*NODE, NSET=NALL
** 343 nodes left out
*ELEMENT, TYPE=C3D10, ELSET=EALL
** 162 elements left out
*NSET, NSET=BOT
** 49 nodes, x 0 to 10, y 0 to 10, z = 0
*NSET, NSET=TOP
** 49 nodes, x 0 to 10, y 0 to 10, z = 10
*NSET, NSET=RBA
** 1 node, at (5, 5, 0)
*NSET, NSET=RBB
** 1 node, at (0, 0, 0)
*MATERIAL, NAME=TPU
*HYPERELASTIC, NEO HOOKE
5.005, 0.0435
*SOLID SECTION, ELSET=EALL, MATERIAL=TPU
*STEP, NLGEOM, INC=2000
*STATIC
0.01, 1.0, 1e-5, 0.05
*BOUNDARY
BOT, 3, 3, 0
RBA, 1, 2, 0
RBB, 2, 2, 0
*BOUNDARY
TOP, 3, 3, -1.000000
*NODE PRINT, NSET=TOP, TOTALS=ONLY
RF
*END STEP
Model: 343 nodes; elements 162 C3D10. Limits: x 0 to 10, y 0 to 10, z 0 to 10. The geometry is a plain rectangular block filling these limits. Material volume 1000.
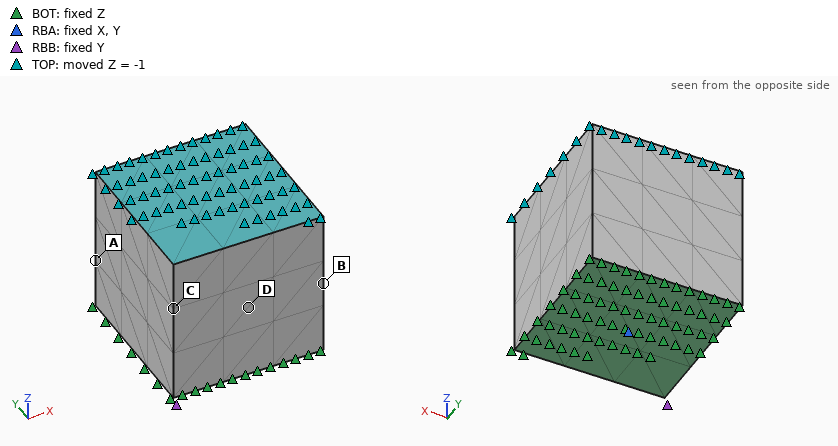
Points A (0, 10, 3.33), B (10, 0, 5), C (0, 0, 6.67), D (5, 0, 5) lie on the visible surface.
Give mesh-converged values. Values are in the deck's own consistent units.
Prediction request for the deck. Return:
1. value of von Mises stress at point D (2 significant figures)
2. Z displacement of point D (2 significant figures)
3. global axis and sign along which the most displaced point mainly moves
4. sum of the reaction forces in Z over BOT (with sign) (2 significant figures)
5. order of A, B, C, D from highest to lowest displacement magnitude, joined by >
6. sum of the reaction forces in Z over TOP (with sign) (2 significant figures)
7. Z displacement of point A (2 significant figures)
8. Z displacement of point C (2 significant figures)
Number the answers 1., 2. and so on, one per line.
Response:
1. 2.9
2. -0.50
3. -Z
4. 310
5. C > B > D > A
6. -310
7. -0.33
8. -0.67
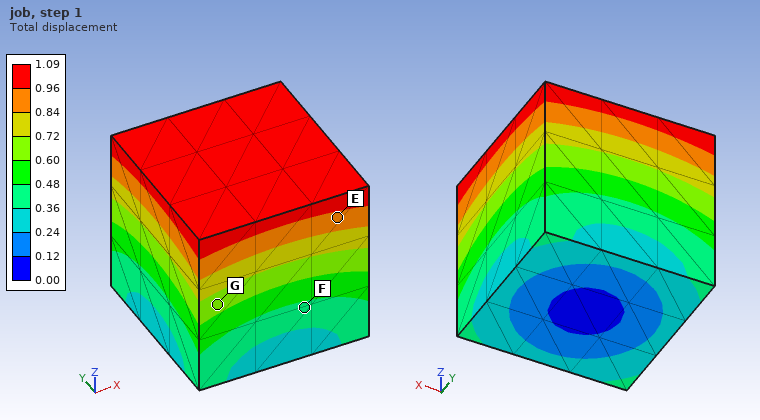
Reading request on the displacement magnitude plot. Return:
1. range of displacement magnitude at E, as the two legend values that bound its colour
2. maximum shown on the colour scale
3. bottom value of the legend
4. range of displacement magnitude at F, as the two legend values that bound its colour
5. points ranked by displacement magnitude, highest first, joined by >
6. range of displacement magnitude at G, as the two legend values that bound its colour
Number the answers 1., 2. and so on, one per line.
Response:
1. 0.84 to 0.96
2. 1.09
3. 0.00
4. 0.36 to 0.48
5. E > G > F
6. 0.60 to 0.72
